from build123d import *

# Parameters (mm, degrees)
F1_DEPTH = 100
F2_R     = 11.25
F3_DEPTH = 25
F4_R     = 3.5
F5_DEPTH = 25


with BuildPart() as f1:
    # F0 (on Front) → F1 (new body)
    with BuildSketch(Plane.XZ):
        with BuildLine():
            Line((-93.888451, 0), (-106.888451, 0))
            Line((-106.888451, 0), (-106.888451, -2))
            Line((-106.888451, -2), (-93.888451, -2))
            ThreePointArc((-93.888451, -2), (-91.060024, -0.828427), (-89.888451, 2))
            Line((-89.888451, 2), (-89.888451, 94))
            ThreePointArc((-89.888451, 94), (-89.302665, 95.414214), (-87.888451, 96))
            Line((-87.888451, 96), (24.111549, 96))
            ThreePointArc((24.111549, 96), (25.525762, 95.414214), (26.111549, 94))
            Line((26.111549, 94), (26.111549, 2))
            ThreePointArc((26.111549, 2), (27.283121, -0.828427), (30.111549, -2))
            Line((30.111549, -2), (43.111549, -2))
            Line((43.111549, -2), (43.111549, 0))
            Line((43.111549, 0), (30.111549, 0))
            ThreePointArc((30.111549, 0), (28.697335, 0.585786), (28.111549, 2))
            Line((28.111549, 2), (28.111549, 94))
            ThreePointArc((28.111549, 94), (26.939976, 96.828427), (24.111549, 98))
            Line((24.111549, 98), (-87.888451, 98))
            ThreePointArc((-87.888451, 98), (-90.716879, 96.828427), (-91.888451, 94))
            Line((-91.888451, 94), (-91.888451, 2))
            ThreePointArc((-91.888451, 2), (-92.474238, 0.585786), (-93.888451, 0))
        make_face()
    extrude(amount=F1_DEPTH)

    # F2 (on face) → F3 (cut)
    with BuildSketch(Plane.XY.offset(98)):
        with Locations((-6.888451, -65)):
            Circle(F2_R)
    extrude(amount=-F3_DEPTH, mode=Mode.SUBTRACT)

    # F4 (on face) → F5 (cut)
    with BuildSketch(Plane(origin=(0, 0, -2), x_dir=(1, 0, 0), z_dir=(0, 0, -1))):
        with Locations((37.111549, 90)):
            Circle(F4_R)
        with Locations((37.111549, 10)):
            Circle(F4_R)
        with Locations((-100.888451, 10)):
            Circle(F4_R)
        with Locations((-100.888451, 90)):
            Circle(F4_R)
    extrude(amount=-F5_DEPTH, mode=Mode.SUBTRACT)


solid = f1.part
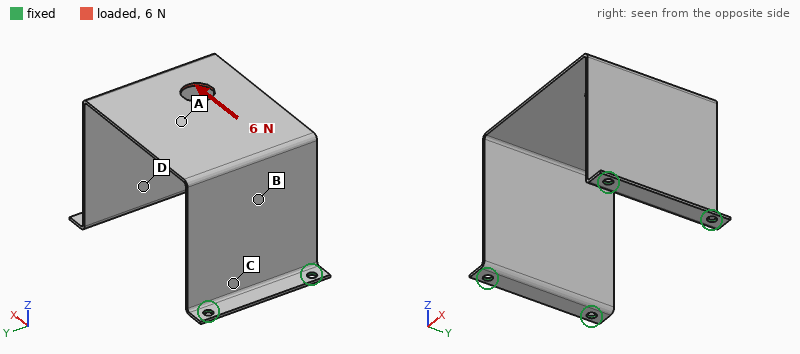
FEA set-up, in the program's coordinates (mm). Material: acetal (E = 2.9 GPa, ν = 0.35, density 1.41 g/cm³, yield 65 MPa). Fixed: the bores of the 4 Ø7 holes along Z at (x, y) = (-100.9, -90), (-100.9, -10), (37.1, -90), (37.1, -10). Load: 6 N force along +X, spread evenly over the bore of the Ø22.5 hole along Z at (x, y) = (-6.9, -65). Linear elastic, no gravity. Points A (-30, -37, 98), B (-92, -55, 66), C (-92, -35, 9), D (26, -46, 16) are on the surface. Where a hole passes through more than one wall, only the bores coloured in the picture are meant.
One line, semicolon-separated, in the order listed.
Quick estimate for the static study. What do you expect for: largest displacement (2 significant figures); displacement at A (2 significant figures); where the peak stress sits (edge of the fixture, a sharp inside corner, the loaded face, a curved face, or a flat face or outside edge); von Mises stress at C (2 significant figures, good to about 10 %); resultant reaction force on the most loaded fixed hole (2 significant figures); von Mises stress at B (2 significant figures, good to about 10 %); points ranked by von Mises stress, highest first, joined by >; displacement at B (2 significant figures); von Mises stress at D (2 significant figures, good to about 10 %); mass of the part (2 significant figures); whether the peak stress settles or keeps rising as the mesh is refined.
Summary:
2.2 mm; 2.2 mm; edge of the fixture; 1.4 MPa; 3.0 N; 0.63 MPa; C > D > B > A; 1.5 mm; 1.1 MPa; 95 g; keeps rising
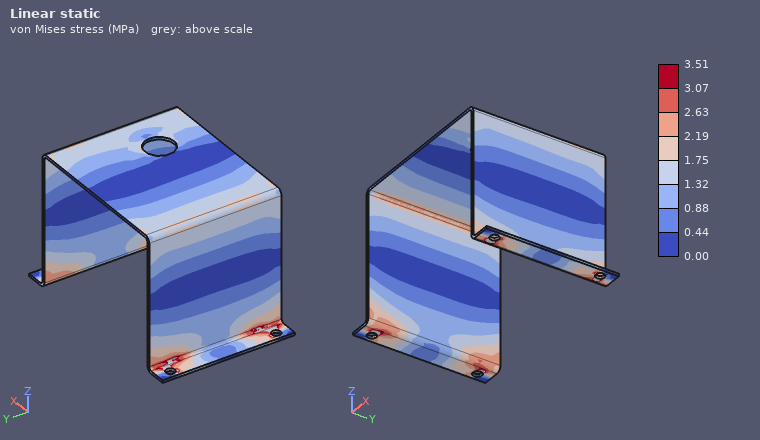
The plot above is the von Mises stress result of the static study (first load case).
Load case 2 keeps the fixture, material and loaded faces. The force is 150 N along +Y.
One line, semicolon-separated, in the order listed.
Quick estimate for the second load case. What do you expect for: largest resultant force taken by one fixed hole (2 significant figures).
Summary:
140 N
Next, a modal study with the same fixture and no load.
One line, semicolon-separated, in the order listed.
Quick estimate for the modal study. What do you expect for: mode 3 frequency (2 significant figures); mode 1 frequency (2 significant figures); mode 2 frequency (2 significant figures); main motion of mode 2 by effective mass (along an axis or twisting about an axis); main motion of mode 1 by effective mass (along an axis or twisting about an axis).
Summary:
210 Hz; 37 Hz; 140 Hz; along Z; along X
